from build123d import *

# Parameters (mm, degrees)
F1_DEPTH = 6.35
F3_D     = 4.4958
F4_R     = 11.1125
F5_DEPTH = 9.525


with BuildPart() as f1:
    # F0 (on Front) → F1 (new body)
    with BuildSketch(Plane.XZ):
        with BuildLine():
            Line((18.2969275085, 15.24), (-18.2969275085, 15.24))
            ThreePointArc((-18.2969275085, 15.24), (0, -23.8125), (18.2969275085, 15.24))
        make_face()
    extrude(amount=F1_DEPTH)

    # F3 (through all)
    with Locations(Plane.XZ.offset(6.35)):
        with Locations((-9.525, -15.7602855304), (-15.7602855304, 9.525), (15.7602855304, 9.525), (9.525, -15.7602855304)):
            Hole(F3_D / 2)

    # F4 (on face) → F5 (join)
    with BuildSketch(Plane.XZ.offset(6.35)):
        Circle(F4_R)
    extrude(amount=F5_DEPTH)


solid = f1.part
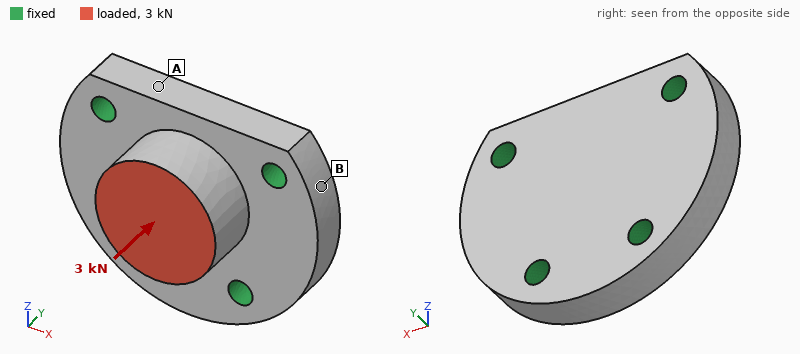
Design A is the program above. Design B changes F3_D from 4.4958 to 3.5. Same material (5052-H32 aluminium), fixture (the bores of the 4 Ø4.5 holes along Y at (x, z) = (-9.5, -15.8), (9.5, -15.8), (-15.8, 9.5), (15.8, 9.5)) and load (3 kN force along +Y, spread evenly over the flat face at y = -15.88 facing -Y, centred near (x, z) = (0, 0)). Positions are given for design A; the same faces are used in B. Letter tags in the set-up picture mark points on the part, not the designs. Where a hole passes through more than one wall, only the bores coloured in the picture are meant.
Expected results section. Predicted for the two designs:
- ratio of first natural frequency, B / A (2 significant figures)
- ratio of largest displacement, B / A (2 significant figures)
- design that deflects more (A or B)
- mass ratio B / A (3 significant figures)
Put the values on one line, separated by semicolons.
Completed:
0.93; 1.1; B; 1.01
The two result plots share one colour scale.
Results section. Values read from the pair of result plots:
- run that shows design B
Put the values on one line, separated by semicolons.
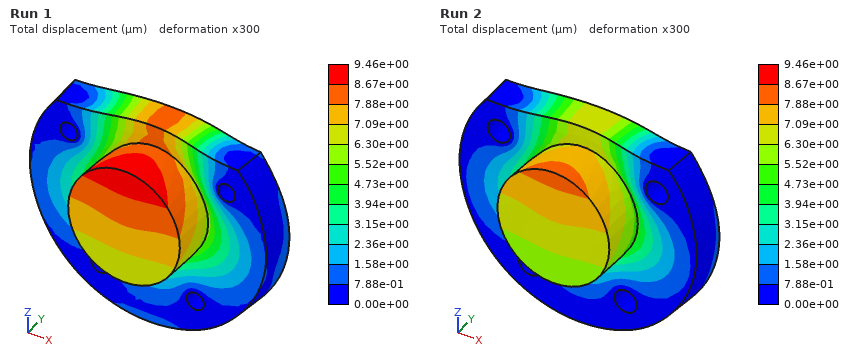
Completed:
Run 1
